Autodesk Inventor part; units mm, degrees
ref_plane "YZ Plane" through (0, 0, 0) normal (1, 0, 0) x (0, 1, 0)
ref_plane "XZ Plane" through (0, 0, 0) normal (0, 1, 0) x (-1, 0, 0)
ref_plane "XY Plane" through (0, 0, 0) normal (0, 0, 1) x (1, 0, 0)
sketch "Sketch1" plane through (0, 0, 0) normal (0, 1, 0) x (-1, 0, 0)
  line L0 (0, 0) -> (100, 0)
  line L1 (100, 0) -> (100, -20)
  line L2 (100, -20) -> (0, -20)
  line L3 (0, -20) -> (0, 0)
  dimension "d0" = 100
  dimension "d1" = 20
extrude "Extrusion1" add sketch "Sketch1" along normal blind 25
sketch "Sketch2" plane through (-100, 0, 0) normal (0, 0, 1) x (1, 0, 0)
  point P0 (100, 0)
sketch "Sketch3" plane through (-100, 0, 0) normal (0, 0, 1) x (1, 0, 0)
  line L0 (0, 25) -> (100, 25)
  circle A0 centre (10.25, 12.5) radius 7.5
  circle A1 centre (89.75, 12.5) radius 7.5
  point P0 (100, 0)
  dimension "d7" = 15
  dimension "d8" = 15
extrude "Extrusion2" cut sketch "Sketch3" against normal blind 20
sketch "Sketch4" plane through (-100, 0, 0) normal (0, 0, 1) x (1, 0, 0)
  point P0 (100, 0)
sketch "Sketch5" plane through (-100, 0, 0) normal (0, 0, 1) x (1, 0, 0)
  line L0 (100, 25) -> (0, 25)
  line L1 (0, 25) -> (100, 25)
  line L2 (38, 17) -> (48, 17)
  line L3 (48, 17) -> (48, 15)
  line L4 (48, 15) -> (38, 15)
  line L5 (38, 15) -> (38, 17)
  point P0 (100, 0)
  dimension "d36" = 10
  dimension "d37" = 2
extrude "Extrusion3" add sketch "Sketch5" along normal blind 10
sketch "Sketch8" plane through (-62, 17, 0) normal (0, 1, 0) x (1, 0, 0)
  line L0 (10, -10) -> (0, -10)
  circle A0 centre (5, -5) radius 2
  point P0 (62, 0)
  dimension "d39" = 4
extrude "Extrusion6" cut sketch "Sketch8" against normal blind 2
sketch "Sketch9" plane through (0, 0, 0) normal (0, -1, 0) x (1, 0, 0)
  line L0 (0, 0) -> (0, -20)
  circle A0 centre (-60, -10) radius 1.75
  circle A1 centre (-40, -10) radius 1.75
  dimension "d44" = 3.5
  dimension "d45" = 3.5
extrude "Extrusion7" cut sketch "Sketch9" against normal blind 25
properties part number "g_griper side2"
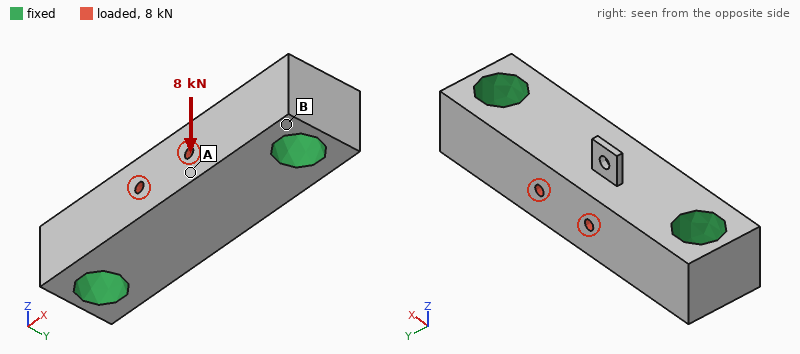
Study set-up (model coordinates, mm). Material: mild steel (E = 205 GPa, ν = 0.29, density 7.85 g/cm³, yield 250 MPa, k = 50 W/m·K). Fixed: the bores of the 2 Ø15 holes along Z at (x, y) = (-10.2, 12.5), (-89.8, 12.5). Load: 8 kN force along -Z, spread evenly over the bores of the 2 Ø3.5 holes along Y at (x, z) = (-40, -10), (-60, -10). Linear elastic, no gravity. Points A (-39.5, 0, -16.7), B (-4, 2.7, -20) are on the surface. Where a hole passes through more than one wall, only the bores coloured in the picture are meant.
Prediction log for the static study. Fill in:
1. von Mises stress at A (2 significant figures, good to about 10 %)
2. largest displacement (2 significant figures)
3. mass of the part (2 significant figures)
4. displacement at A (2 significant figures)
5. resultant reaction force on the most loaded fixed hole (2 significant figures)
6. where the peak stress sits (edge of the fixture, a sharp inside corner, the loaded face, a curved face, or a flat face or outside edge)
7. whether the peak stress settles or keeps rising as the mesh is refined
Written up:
16 MPa
6.4 µm
330 g
5.5 µm
4.0 kN
edge of the fixture
keeps rising
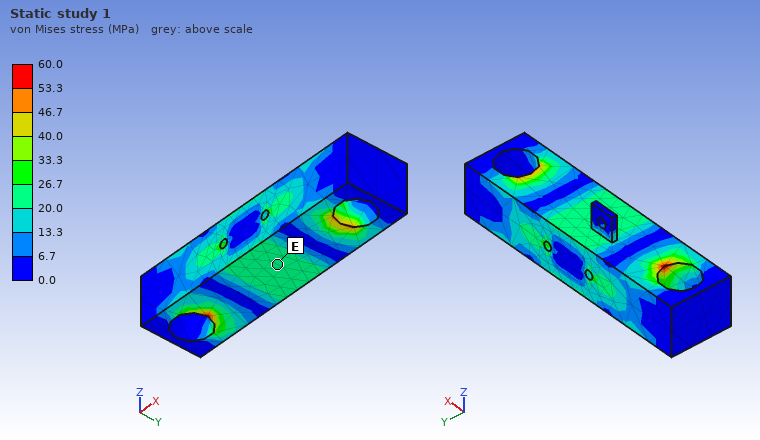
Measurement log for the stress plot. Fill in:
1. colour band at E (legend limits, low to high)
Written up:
20.0 to 26.7 MPa
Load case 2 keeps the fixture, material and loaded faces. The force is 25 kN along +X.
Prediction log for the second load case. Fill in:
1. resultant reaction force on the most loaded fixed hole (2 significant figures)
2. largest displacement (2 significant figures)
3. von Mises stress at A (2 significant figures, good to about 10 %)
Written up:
13 kN
4.1 µm
12 MPa
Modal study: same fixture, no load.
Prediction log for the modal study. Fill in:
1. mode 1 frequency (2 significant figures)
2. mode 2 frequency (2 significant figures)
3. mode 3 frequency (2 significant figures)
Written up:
14 kHz
15 kHz
16 kHz
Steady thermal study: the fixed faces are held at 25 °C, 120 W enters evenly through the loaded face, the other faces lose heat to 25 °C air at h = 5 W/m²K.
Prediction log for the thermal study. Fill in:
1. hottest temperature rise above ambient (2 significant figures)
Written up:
67 K
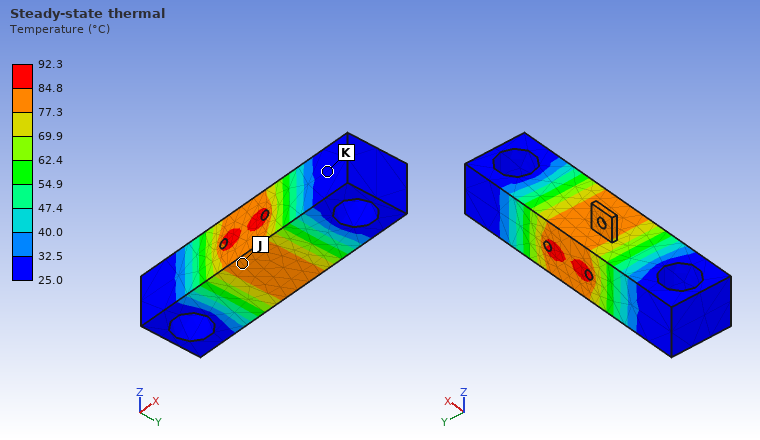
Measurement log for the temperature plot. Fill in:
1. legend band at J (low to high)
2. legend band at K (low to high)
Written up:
77.3 to 84.8 °C
25.0 to 32.5 °C
